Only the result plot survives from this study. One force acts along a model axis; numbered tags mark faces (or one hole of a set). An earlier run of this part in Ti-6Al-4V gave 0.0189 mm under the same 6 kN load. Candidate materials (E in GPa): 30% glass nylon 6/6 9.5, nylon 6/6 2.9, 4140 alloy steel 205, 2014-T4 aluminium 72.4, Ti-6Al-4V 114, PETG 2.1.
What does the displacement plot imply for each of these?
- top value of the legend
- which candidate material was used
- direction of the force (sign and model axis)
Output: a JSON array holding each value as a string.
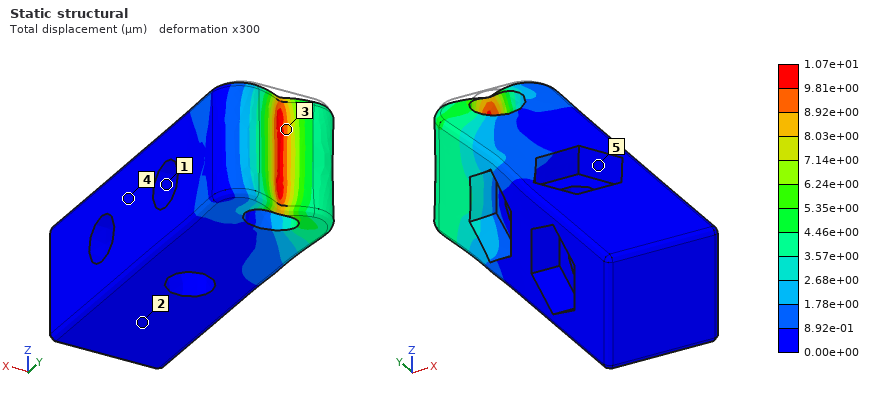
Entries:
["1.07e+01 µm", "4140 alloy steel", "-Y"]
